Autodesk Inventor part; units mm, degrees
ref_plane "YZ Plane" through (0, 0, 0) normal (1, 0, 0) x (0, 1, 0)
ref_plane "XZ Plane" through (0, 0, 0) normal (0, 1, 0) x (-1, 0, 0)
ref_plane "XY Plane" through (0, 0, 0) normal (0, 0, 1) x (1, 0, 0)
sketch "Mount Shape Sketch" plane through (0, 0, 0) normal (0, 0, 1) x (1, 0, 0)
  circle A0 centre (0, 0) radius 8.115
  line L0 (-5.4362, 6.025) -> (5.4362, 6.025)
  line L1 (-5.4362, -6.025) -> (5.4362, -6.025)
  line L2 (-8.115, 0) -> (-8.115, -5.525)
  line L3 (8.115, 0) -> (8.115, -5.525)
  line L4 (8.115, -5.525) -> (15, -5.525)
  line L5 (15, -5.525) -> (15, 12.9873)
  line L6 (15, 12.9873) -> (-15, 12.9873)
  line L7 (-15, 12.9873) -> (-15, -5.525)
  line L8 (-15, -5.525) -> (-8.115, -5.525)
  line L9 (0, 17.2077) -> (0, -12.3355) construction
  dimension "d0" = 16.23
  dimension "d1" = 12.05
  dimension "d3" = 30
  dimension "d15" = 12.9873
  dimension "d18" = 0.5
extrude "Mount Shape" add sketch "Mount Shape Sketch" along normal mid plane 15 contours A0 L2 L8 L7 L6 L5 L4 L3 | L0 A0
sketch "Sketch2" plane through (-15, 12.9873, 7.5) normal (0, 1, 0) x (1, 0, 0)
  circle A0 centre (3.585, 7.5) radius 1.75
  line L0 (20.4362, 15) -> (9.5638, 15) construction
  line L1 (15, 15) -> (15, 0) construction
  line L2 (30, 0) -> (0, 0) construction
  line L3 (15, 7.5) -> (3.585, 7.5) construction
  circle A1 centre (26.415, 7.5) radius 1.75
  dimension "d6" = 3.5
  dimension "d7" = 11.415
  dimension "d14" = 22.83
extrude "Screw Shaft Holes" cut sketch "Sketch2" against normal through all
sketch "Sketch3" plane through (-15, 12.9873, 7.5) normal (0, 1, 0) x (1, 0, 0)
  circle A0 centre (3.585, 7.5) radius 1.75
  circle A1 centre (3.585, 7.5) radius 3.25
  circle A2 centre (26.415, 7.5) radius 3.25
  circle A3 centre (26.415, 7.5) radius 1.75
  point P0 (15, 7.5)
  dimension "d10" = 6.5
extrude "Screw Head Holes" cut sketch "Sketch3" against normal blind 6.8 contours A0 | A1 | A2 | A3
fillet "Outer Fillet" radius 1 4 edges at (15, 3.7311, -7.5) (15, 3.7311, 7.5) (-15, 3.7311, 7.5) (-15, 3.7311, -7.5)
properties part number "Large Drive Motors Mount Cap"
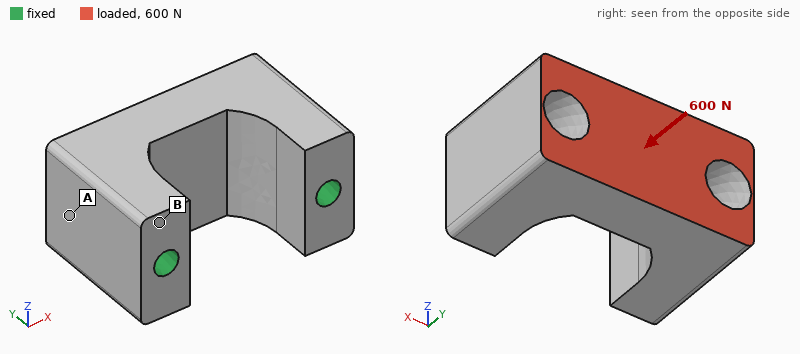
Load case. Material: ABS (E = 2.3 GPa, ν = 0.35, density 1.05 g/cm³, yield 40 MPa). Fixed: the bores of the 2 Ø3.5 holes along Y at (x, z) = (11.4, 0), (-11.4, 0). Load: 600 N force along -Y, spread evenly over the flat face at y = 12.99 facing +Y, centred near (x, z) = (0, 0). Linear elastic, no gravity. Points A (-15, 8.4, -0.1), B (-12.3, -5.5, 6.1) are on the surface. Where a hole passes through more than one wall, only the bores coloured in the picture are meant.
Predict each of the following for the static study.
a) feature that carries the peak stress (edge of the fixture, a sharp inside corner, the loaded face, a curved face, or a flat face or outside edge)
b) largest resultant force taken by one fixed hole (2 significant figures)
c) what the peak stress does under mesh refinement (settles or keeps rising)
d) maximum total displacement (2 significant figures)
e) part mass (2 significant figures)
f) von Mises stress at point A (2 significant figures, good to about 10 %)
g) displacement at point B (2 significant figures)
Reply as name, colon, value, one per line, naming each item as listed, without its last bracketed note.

feature that carries the peak stress: edge of the fixture
largest resultant force taken by one fixed hole: 320 N
what the peak stress does under mesh refinement: keeps rising
maximum total displacement: 35 µm
part mass: 5.2 g
von Mises stress at point A: 2.9 MPa
displacement at point B: 7.4 µm
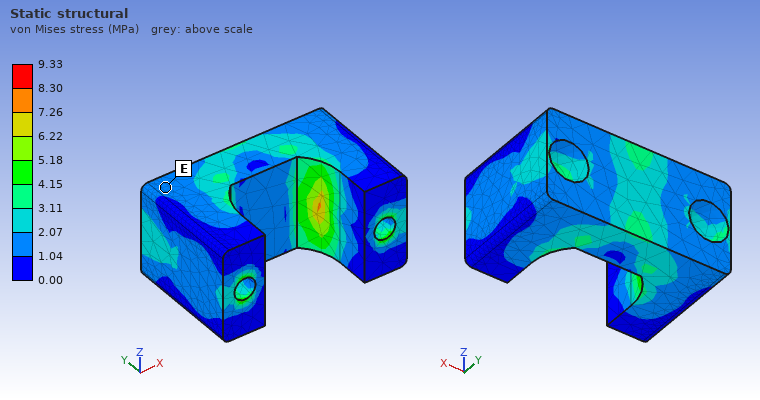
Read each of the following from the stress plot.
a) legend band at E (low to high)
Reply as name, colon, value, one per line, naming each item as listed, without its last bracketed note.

legend band at E: 1.04 to 2.07 MPa
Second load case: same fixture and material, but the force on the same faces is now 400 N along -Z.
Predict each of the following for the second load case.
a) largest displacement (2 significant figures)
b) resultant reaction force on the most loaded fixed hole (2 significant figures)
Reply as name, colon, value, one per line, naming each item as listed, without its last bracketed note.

largest displacement: 0.11 mm
resultant reaction force on the most loaded fixed hole: 200 N
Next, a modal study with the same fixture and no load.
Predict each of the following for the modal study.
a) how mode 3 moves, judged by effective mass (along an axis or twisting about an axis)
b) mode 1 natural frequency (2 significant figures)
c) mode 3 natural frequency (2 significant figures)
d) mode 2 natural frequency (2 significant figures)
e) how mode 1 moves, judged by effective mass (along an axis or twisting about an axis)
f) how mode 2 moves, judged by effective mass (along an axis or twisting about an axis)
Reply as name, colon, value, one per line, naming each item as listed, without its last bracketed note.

how mode 3 moves, judged by effective mass: twisting about Y
mode 1 natural frequency: 8200 Hz
mode 3 natural frequency: 13 kHz
mode 2 natural frequency: 12 kHz
how mode 1 moves, judged by effective mass: along Z
how mode 2 moves, judged by effective mass: along X
